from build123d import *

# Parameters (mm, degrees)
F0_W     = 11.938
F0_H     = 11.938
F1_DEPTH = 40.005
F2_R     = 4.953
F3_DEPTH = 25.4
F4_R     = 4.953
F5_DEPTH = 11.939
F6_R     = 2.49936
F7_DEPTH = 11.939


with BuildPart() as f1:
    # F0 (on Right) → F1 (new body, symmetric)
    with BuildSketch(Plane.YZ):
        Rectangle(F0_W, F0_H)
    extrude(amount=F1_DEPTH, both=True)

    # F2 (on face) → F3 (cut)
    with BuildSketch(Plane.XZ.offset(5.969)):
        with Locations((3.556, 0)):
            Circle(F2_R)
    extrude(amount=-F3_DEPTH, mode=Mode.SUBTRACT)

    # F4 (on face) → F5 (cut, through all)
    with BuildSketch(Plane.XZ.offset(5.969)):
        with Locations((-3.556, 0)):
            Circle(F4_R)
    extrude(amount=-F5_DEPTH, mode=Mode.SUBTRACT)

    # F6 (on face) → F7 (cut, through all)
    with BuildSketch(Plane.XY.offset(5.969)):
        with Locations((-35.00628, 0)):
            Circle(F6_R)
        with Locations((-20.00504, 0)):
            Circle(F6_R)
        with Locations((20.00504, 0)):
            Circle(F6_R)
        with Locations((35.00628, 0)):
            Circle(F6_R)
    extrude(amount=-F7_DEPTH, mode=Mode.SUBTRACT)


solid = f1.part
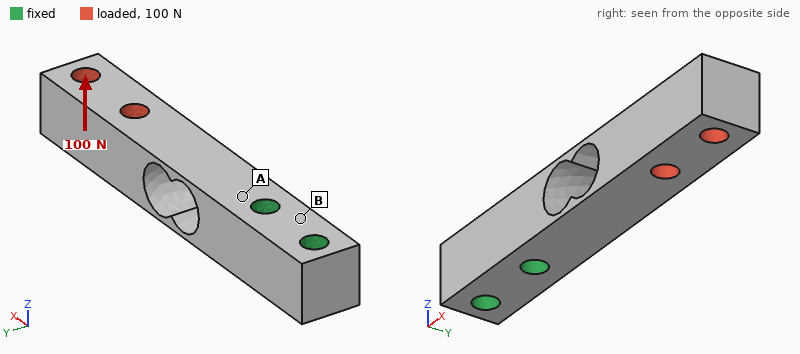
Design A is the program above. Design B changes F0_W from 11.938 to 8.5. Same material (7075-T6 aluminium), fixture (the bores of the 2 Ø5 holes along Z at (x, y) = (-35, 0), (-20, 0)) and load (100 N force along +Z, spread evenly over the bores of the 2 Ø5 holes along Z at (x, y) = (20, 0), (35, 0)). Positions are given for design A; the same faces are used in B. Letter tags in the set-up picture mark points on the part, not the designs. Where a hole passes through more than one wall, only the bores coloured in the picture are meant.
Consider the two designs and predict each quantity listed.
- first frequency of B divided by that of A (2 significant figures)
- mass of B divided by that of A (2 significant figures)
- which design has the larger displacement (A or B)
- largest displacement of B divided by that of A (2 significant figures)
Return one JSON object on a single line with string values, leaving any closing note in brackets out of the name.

{"first frequency of B divided by that of A": "0.94", "mass of B divided by that of A": "0.68", "which design has the larger displacement": "B", "largest displacement of B divided by that of A": "1.5"}
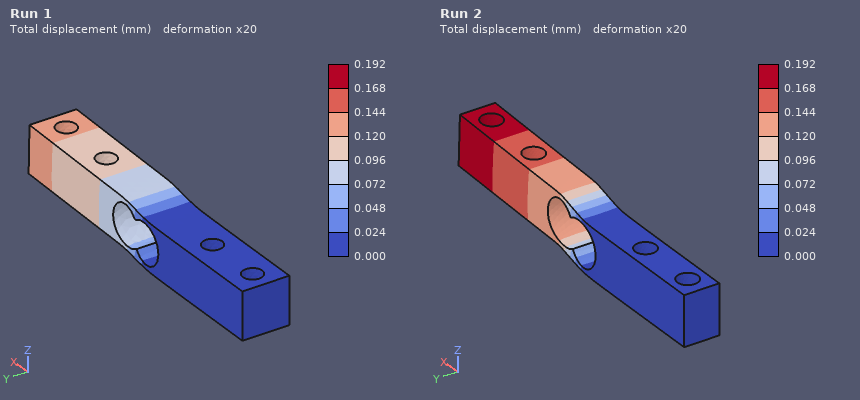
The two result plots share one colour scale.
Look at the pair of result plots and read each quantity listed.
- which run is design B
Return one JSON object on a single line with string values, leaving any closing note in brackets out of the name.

{"which run is design B": "Run 2"}
